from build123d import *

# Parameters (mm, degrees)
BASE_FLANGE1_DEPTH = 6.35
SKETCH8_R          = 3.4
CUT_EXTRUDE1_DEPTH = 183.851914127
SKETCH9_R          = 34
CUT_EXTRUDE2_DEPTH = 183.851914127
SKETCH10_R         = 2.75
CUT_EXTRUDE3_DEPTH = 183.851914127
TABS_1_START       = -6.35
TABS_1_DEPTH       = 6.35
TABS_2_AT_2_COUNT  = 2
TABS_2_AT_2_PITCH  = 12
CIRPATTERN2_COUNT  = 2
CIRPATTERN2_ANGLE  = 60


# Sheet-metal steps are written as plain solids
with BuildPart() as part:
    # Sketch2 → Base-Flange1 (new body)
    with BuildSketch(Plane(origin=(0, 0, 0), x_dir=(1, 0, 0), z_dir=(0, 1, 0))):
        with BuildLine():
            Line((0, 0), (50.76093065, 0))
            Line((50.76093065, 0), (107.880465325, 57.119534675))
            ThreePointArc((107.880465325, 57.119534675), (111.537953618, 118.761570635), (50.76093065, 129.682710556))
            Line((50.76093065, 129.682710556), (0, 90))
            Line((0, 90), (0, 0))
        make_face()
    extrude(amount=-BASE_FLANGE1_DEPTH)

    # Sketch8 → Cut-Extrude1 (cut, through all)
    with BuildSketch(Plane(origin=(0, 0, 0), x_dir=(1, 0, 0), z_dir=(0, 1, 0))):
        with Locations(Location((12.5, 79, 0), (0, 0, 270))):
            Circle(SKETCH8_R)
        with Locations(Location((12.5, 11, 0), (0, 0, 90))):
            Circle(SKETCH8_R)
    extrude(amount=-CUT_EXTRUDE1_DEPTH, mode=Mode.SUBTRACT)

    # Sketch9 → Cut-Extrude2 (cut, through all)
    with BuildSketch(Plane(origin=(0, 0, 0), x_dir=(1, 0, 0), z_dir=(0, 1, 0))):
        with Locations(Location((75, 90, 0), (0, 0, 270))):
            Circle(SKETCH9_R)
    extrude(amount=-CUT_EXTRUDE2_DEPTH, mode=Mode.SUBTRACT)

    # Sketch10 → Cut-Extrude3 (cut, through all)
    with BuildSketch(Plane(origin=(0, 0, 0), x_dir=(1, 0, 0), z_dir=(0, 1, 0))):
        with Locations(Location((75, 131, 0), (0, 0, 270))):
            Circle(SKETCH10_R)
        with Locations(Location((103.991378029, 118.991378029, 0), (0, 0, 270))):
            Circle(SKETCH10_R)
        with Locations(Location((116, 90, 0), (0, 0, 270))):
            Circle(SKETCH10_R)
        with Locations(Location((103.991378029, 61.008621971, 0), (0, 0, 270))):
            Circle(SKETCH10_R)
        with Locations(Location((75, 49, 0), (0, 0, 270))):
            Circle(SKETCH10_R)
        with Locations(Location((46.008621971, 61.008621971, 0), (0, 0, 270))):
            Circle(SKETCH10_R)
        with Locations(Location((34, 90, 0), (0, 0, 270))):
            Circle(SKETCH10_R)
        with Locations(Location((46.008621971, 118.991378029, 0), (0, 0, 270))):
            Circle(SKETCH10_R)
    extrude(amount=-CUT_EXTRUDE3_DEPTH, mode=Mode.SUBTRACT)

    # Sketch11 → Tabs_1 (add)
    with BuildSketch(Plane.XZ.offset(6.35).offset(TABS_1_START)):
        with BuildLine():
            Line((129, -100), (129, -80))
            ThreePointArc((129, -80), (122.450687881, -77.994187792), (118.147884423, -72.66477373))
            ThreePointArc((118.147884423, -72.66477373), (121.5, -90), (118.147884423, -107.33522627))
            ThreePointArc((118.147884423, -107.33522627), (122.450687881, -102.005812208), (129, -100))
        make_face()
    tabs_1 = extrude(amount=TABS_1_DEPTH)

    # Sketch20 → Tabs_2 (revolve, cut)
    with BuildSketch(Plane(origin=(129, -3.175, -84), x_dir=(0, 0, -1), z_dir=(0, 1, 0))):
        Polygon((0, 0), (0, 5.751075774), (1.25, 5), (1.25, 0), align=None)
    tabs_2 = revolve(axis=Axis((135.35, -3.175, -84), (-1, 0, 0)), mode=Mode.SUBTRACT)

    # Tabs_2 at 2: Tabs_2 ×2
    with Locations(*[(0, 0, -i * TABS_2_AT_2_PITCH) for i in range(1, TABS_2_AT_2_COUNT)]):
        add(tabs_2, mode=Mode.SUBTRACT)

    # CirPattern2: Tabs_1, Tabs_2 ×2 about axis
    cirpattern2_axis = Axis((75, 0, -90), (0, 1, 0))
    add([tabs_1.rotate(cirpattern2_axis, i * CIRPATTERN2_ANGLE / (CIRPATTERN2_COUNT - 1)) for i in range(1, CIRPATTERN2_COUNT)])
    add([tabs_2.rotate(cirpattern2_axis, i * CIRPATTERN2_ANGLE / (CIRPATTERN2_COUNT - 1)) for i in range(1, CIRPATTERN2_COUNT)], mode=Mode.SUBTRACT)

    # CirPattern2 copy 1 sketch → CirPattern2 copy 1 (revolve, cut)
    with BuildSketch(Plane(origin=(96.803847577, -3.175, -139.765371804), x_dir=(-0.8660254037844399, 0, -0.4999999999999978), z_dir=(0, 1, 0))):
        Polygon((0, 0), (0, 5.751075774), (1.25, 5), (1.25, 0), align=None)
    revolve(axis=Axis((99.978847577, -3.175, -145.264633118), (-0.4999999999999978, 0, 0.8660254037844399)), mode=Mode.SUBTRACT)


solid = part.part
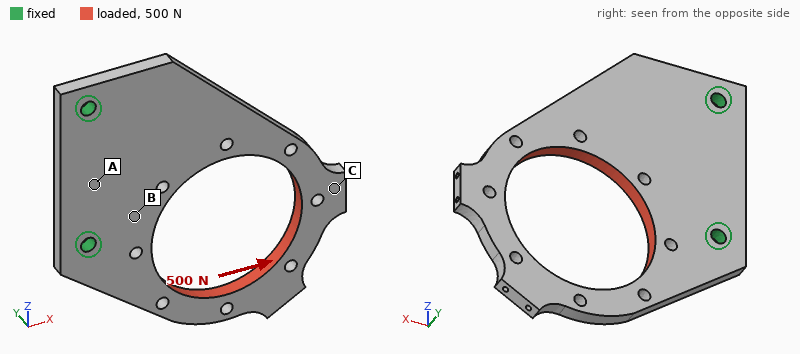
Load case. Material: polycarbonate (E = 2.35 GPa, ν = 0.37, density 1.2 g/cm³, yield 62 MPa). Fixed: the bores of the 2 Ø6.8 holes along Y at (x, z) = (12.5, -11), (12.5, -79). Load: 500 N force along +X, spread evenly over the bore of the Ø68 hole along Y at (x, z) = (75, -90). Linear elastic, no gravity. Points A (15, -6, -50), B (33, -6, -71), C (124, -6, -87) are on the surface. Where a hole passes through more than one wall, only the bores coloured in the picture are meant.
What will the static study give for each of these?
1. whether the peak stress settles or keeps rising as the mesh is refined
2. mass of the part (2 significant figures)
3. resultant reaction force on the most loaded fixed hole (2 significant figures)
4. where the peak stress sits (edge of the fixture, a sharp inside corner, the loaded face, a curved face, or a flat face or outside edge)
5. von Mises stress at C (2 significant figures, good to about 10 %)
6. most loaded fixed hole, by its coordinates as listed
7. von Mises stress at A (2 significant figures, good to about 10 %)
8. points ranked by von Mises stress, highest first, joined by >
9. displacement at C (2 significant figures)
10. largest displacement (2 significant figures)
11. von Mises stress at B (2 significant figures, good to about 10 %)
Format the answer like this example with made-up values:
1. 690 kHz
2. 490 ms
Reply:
1. keeps rising
2. 66 g
3. 560 N
4. edge of the fixture
5. 1.7 MPa
6. (12.5, -79)
7. 0.82 MPa
8. B > C > A
9. 0.60 mm
10. 0.68 mm
11. 3.0 MPa
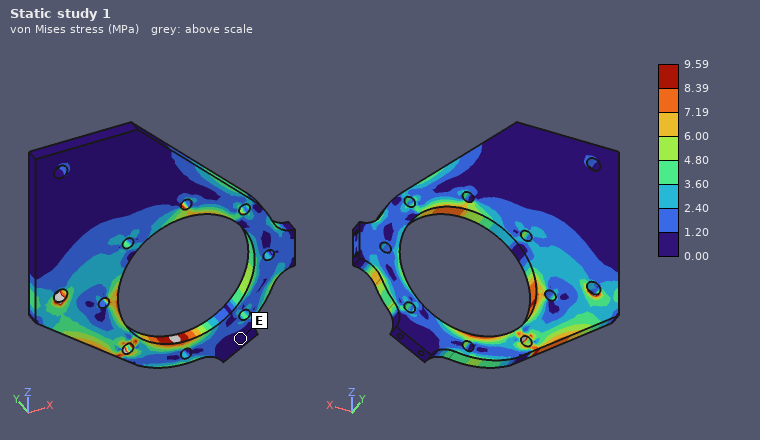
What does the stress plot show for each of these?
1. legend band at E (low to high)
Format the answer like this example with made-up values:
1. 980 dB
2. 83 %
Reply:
1. 0.00 to 1.20 MPa
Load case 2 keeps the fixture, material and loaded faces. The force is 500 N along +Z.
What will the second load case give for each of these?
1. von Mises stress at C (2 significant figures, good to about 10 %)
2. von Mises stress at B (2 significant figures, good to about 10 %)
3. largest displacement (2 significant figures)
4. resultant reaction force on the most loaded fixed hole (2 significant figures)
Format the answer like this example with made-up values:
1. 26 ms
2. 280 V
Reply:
1. 1.6 MPa
2. 3.8 MPa
3. 0.76 mm
4. 510 N
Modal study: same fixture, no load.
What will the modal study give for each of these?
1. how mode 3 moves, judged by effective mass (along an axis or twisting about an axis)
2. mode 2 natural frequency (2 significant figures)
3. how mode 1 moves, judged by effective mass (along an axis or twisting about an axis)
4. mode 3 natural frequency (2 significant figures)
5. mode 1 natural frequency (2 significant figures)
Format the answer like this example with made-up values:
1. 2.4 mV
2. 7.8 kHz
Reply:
1. along Y
2. 270 Hz
3. along Y
4. 500 Hz
5. 120 Hz
